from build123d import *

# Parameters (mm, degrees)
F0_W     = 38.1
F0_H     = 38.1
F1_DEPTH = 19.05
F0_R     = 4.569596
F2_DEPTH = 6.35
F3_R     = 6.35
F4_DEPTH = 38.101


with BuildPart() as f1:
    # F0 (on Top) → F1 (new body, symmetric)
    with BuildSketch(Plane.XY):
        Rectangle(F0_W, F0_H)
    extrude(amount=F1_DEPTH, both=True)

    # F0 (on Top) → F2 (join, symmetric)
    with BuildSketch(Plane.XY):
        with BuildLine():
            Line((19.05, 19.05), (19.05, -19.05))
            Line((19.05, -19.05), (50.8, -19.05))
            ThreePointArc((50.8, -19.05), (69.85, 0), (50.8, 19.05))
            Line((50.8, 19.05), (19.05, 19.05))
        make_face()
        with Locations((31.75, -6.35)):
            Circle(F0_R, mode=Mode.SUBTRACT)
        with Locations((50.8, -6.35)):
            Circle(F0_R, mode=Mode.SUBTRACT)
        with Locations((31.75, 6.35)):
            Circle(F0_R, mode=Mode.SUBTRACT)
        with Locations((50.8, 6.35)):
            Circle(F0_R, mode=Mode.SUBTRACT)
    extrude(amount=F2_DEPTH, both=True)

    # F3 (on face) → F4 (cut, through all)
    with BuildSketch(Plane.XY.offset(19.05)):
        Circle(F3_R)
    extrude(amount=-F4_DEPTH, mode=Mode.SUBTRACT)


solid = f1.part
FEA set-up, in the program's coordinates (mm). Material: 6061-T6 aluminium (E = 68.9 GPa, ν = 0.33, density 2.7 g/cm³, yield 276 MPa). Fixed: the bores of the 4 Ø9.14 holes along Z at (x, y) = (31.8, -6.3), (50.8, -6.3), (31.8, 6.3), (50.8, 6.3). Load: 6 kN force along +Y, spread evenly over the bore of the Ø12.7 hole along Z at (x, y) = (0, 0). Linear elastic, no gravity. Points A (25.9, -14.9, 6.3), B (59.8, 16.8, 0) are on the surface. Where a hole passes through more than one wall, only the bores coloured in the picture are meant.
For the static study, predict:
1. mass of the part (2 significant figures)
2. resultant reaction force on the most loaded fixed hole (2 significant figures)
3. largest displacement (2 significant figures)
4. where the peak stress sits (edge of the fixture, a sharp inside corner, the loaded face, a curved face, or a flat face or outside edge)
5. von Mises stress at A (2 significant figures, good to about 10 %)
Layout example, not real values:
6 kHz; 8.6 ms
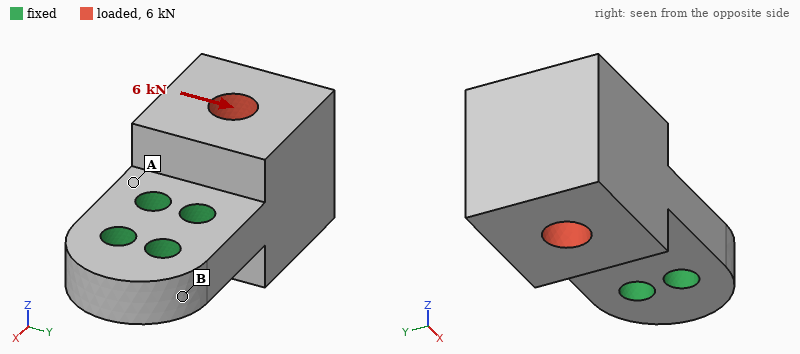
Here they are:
190 g; 7.4 kN; 51 µm; edge of the fixture; 32 MPa
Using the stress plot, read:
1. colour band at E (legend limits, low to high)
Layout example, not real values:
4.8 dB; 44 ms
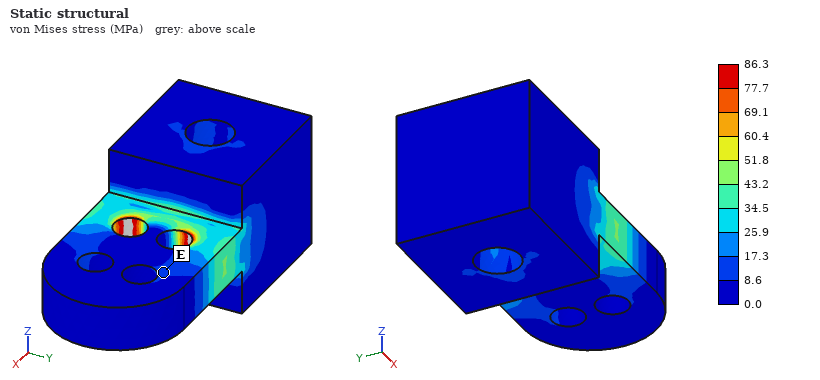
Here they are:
8.6 to 17.3 MPa
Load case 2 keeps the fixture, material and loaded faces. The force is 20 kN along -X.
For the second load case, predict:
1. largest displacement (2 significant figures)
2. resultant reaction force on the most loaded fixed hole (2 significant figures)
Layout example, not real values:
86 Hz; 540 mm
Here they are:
19 µm; 9.4 kN
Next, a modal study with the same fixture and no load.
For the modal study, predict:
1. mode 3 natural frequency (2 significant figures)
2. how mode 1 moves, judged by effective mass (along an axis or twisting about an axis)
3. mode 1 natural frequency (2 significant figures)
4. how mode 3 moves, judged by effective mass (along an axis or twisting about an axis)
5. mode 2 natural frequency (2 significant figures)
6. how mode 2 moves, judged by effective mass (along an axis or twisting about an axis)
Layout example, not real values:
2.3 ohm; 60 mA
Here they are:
7000 Hz; along Z; 2700 Hz; twisting about X; 5400 Hz; along Y
